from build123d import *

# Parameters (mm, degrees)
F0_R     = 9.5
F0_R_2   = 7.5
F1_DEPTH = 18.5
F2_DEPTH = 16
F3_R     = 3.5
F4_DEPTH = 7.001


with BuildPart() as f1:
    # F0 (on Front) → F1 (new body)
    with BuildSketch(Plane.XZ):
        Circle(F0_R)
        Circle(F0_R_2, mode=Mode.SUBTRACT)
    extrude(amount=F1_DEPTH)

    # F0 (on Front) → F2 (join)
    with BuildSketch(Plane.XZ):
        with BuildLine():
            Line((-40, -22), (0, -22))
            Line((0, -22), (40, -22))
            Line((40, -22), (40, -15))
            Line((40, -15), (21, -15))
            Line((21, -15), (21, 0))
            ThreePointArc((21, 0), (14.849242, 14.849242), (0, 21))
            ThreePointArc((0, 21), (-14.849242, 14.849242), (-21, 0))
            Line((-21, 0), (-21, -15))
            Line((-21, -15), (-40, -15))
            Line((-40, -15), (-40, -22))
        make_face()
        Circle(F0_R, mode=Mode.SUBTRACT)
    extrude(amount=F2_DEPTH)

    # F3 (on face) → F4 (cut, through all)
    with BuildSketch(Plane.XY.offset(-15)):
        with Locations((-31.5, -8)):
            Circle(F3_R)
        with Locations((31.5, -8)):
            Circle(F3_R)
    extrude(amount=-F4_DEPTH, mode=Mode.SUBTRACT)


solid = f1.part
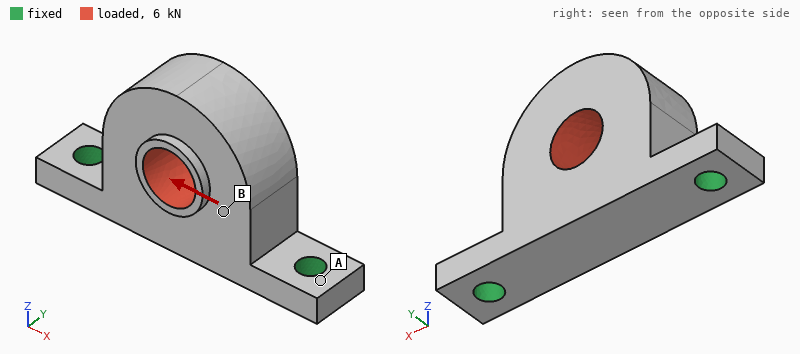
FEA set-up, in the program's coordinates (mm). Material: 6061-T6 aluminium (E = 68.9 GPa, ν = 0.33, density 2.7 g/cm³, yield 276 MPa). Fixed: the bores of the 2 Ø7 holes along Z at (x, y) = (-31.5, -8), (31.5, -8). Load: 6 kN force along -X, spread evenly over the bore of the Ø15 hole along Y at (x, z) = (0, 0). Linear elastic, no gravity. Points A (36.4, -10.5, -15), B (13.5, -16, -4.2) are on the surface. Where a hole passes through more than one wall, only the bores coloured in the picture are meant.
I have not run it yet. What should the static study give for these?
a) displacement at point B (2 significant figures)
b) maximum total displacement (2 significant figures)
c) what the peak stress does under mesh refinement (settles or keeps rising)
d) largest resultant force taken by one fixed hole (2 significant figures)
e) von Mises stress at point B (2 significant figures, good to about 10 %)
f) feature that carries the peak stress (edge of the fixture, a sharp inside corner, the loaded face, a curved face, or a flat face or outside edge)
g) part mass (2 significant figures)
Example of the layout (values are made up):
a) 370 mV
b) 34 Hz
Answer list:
a) 23 µm
b) 46 µm
c) keeps rising
d) 3.7 kN
e) 26 MPa
f) edge of the fixture
g) 73 g
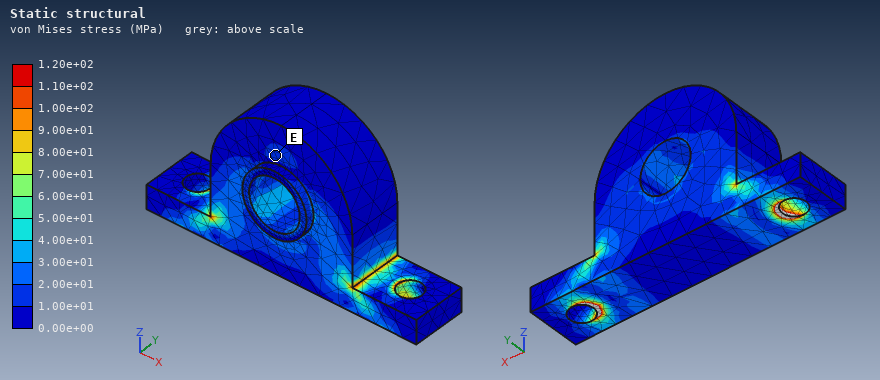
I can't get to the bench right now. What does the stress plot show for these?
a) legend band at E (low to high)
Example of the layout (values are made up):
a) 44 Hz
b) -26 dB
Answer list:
a) 1.00e+01 to 2.00e+01 MPa
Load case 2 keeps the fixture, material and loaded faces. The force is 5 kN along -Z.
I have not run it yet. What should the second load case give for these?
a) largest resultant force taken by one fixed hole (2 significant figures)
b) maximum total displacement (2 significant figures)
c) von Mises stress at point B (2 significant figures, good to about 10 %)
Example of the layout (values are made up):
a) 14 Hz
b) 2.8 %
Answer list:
a) 2.8 kN
b) 50 µm
c) 16 MPa
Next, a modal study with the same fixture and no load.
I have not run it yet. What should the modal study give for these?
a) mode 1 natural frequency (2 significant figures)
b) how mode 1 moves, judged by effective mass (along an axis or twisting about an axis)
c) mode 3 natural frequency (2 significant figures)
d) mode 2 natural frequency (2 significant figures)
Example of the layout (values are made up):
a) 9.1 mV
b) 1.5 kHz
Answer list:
a) 2600 Hz
b) along Y
c) 8700 Hz
d) 8700 Hz
